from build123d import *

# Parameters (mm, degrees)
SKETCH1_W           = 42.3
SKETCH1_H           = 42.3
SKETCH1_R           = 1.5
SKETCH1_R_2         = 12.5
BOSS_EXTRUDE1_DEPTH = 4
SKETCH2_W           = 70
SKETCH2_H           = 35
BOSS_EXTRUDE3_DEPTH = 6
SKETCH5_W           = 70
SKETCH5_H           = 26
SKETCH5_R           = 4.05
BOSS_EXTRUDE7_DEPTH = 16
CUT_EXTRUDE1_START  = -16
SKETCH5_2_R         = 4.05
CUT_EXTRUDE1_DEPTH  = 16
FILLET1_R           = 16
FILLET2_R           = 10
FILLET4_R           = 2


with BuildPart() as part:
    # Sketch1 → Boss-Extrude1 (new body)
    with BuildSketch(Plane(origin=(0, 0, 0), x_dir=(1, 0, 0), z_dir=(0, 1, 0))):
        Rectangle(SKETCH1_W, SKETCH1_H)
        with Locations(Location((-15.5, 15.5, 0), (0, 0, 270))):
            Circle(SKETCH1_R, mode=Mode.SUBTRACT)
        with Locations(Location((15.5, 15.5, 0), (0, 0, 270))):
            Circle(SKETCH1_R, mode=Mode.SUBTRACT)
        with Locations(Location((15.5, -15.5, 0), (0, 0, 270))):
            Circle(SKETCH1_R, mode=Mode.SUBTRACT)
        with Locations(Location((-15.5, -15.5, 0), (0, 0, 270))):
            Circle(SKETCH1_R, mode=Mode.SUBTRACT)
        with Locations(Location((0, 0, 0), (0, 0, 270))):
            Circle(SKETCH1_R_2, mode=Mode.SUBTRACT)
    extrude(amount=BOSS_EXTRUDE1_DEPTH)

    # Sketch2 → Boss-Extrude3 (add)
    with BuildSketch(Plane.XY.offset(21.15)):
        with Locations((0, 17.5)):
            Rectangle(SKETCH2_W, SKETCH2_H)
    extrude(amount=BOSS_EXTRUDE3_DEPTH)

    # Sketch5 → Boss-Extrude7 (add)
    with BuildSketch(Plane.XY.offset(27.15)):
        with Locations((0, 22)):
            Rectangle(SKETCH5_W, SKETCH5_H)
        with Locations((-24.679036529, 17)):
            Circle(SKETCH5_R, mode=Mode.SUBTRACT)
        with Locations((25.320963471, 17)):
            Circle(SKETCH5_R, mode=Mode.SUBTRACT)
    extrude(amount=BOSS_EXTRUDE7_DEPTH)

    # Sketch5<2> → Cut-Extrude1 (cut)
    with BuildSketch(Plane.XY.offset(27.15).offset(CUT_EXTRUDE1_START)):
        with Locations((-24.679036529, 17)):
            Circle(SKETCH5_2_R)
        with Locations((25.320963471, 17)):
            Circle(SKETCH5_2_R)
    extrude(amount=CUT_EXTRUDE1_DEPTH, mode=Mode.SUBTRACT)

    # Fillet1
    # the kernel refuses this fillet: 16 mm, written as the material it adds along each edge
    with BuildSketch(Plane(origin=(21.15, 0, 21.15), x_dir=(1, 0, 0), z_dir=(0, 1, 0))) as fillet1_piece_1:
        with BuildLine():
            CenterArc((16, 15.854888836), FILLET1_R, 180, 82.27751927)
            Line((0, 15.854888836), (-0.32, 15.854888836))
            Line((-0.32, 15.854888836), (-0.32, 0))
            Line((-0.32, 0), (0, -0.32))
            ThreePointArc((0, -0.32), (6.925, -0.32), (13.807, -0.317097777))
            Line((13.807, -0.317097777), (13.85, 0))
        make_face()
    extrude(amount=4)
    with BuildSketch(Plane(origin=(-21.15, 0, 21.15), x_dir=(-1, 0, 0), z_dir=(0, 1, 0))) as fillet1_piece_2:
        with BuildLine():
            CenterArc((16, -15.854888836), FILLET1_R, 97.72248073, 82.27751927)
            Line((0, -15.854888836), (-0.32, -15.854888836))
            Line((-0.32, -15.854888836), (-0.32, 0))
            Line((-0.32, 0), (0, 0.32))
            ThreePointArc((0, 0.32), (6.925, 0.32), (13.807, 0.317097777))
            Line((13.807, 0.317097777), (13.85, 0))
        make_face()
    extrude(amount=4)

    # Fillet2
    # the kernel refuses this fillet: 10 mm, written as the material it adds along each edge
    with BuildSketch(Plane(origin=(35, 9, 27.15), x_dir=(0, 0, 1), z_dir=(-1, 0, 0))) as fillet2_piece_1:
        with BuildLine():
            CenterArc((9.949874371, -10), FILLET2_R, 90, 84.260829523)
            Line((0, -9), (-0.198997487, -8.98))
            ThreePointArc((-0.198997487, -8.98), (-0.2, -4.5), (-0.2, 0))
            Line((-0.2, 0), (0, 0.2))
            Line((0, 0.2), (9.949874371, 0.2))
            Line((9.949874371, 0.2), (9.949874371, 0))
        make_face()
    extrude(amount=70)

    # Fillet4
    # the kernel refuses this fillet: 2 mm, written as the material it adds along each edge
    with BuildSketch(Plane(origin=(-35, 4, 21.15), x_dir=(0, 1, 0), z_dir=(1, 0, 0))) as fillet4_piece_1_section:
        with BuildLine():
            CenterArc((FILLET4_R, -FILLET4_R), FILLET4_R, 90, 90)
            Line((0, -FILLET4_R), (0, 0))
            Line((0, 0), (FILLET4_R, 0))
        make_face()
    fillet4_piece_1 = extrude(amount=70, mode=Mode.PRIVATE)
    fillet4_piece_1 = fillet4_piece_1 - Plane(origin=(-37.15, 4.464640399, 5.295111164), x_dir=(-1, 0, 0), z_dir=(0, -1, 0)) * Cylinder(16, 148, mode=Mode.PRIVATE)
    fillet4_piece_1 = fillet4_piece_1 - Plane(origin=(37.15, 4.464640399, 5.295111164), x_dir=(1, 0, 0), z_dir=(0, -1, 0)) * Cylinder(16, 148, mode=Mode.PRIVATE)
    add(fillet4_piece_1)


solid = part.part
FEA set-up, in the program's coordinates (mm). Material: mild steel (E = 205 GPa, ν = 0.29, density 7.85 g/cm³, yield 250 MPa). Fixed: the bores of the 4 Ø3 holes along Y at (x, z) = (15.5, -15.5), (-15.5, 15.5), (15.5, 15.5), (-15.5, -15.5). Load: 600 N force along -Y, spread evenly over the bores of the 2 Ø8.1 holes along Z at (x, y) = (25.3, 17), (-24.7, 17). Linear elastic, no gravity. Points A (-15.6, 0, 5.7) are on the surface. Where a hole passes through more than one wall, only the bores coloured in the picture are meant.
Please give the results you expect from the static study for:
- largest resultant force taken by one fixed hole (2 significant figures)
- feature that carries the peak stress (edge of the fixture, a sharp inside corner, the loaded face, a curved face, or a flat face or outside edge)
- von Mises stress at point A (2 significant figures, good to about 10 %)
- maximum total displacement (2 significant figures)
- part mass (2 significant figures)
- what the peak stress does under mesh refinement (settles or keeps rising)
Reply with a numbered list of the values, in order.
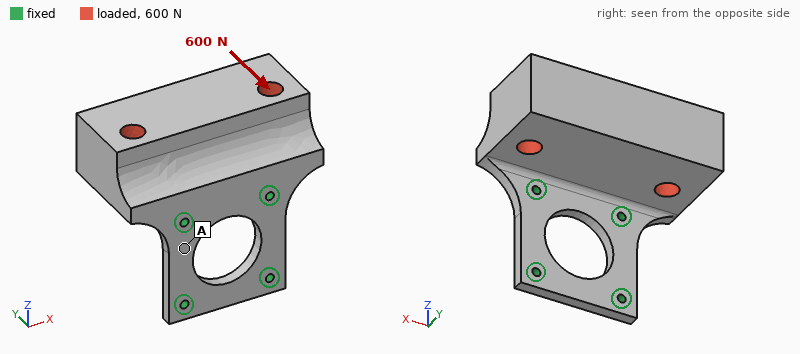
1. 330 N
2. edge of the fixture
3. 15 MPa
4. 56 µm
5. 380 g
6. keeps rising
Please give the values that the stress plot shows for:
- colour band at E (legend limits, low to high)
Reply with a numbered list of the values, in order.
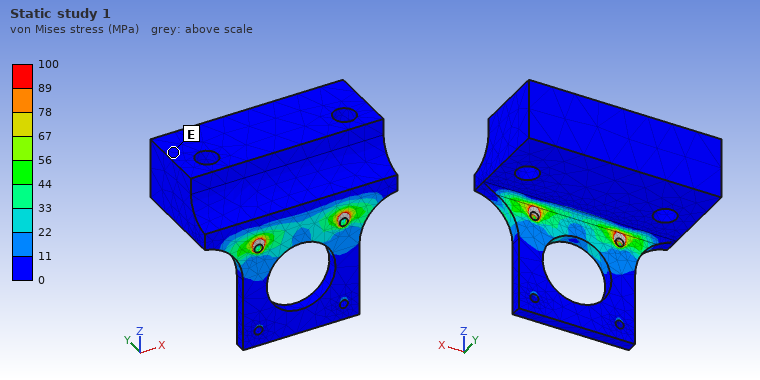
1. 0 to 11 MPa
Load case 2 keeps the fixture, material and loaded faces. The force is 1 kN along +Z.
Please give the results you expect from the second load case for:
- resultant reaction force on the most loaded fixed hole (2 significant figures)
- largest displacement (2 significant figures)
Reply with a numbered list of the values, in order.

1. 470 N
2. 99 µm
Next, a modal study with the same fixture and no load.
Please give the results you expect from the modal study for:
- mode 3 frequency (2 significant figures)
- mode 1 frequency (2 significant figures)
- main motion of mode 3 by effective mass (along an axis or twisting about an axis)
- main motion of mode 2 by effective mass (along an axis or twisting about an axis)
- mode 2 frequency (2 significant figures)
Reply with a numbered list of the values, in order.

1. 5400 Hz
2. 860 Hz
3. along X
4. along X
5. 3100 Hz
